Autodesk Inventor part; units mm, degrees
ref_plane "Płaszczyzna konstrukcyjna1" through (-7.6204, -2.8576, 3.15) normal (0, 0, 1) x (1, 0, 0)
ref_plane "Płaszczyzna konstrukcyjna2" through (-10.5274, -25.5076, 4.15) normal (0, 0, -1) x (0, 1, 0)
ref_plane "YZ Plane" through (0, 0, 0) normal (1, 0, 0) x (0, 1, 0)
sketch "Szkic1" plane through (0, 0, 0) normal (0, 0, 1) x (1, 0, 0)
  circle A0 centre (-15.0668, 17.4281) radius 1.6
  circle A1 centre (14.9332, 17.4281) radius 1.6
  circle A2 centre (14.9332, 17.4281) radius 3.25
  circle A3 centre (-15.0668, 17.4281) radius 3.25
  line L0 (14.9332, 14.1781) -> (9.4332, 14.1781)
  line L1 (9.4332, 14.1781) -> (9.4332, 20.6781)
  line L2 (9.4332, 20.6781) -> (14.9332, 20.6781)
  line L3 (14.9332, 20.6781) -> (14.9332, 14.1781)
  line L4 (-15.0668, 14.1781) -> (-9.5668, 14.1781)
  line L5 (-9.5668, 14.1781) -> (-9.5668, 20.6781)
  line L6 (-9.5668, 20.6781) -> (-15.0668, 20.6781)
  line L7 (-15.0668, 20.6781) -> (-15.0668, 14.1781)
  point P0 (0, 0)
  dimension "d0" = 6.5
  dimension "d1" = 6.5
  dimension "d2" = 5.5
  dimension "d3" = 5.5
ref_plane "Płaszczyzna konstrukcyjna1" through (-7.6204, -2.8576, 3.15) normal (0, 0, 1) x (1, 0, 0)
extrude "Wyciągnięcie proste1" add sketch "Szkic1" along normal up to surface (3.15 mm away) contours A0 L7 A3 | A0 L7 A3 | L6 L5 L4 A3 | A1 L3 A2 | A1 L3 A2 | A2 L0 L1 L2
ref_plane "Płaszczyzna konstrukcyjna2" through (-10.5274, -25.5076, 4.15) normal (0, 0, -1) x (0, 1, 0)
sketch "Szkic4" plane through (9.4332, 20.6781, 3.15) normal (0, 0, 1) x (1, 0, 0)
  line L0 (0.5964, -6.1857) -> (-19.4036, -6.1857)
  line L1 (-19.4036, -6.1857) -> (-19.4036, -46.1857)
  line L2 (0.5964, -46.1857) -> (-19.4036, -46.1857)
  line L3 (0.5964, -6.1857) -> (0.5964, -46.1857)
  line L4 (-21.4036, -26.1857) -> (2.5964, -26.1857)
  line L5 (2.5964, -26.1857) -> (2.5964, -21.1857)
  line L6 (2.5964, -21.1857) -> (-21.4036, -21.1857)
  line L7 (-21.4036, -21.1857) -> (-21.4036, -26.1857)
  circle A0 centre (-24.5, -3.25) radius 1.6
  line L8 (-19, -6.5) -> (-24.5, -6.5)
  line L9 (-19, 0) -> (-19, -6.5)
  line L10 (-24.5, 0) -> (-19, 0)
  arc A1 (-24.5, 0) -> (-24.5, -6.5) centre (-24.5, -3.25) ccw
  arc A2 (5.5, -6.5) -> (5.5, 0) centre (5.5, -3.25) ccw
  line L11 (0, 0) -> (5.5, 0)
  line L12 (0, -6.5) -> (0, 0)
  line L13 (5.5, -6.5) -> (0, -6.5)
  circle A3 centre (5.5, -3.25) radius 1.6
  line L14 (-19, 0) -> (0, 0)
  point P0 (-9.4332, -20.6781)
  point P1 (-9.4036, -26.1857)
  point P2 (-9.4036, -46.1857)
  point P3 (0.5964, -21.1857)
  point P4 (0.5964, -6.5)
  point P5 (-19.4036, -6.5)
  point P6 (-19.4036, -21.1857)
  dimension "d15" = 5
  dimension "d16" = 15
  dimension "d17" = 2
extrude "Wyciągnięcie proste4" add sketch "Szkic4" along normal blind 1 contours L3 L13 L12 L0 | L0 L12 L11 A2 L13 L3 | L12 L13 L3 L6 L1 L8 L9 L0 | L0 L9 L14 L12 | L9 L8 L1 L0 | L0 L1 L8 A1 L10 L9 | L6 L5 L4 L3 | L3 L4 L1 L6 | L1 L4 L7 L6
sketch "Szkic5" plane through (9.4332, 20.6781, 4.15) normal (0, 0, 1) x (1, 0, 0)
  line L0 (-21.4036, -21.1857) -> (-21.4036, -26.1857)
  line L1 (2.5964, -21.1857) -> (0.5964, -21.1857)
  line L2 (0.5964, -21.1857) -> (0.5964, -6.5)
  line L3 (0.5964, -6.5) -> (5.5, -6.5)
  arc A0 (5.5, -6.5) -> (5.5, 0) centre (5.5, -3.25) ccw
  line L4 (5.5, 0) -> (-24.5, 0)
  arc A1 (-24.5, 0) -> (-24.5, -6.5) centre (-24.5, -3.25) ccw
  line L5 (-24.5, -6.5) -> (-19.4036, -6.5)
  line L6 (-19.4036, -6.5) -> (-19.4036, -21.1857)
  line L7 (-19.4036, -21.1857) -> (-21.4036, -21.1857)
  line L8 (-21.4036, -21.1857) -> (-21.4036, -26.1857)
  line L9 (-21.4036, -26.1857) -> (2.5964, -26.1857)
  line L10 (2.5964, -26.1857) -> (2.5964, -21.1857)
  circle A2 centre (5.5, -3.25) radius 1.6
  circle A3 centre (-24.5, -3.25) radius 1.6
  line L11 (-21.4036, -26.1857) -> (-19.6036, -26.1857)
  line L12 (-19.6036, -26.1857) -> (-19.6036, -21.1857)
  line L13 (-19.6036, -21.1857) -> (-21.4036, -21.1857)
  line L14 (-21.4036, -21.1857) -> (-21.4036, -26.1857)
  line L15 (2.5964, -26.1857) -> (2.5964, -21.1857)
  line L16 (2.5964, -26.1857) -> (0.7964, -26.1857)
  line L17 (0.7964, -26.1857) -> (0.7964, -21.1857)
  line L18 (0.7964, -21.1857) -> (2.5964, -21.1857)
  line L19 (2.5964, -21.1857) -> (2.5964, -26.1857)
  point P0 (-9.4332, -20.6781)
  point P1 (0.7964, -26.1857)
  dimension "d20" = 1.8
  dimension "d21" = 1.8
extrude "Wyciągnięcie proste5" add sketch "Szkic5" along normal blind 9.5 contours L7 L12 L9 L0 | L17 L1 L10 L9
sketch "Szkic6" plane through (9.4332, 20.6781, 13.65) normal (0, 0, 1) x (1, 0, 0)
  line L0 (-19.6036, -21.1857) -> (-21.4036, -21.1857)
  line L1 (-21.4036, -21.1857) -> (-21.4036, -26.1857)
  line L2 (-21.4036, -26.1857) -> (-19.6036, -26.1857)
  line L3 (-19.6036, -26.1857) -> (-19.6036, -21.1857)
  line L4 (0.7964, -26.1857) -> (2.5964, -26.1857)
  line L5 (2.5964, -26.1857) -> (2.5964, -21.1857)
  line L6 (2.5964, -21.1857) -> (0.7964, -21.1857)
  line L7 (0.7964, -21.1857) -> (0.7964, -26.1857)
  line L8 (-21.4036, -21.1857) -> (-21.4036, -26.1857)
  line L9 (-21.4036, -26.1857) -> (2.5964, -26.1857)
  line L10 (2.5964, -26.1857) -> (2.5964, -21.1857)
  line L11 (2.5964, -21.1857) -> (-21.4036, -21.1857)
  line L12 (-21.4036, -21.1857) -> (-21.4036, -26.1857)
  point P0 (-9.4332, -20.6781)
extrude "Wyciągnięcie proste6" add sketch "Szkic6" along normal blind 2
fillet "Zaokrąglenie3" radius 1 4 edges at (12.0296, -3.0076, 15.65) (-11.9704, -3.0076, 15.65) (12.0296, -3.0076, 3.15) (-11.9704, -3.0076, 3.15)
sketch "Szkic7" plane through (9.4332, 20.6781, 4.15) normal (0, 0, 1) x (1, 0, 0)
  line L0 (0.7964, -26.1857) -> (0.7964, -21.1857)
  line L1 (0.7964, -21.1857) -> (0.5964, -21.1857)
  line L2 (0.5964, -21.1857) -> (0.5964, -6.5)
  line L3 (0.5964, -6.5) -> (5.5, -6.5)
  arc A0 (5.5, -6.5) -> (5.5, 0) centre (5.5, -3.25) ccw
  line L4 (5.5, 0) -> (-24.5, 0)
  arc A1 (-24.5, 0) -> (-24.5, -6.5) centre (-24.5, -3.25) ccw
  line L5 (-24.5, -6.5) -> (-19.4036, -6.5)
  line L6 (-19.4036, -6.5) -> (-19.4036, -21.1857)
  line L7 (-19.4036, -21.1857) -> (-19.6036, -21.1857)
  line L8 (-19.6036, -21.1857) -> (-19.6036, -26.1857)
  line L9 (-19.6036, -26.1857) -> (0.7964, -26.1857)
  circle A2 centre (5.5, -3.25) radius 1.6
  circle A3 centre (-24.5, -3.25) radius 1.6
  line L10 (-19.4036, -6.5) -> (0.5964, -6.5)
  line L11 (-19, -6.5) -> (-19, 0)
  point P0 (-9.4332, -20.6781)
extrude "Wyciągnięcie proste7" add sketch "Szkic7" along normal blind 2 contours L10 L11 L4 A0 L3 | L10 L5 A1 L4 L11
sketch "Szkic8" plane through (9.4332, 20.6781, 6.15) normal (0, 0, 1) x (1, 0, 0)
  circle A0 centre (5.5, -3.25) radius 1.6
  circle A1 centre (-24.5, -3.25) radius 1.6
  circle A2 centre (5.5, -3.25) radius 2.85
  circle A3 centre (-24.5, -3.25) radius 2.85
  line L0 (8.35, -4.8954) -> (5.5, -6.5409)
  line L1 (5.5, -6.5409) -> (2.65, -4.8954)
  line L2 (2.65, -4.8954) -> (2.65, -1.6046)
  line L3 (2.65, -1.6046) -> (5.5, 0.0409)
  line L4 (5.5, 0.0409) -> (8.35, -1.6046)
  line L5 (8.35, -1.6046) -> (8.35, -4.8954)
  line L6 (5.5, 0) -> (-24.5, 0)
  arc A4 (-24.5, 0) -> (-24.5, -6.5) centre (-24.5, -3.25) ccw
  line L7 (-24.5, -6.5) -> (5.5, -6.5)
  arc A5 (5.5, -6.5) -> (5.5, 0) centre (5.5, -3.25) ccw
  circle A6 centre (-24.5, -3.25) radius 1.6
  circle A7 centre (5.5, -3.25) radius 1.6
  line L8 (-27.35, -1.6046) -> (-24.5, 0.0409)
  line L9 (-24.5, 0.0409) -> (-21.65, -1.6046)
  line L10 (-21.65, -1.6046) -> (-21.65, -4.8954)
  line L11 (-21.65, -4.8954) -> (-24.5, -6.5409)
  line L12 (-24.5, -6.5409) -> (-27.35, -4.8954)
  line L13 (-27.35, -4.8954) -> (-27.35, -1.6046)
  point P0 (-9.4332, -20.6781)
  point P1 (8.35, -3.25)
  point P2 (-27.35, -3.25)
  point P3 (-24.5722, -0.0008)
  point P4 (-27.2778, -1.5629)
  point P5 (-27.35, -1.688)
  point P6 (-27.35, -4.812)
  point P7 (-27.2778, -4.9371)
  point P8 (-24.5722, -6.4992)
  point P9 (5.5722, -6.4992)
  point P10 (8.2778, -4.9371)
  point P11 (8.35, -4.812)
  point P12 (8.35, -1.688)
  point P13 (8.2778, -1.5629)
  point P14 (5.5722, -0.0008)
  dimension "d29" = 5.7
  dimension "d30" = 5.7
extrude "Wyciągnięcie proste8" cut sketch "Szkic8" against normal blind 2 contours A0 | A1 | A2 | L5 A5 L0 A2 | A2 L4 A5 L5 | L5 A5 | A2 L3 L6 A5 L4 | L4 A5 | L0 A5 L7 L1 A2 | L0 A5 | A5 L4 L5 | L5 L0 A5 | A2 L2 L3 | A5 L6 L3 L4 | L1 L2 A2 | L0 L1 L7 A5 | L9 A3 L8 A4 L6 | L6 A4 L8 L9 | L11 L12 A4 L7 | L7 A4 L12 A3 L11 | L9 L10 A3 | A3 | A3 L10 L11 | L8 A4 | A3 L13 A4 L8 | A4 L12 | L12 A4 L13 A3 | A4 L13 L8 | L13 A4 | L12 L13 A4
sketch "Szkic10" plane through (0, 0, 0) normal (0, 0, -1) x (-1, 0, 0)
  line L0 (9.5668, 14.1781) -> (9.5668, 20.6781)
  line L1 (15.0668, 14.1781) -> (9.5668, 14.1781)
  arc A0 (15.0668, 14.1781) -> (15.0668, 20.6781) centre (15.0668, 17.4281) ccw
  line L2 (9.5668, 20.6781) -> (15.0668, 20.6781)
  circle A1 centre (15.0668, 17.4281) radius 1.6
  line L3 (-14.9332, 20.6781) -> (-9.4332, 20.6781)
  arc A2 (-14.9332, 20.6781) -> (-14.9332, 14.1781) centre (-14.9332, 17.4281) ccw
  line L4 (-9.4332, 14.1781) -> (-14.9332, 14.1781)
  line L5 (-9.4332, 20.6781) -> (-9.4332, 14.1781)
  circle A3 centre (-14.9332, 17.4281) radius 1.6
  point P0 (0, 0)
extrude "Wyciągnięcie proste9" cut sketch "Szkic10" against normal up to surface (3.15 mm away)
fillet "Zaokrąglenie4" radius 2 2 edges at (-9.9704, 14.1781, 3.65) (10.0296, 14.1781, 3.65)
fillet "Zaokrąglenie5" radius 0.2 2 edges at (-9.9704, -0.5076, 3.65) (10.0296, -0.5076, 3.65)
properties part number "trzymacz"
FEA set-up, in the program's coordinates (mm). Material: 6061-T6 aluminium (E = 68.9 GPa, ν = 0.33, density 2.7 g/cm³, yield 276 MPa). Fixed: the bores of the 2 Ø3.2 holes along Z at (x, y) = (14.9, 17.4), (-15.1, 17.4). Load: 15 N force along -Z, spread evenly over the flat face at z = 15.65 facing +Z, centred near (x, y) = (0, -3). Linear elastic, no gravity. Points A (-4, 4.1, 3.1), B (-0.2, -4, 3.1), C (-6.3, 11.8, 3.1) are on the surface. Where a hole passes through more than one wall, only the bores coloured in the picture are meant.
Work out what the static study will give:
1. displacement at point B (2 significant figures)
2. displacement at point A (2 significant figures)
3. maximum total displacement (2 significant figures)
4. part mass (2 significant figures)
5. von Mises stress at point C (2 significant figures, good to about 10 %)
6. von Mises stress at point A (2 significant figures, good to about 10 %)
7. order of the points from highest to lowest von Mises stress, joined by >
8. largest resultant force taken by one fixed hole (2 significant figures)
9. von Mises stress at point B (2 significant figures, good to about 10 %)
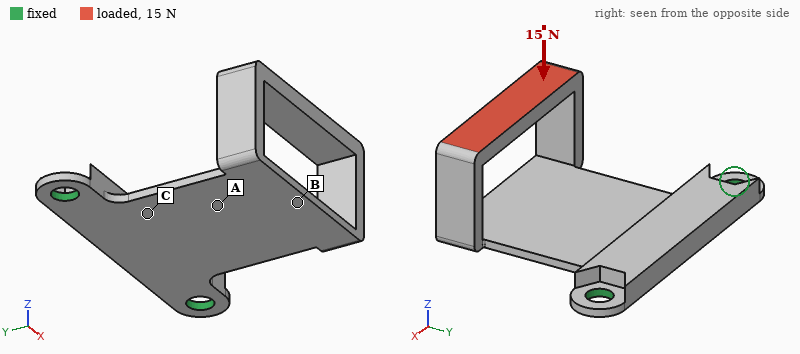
0.29 mm
0.13 mm
0.43 mm
3.7 g
60 MPa
28 MPa
C > A > B
26 N
9.6 MPa
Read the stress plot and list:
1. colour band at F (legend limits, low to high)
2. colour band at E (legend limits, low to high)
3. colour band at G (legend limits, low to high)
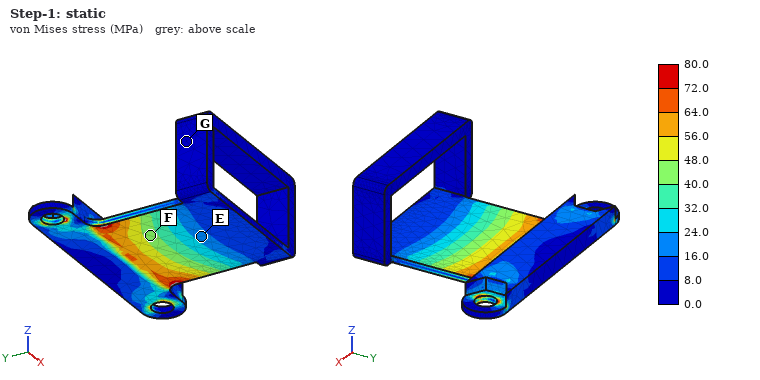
40.0 to 48.0 MPa
16.0 to 24.0 MPa
0.0 to 8.0 MPa
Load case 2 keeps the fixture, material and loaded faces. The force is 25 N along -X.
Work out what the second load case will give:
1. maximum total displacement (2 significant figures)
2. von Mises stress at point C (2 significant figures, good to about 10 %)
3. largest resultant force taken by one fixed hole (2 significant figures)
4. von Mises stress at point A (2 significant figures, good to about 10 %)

0.31 mm
50 MPa
25 N
49 MPa
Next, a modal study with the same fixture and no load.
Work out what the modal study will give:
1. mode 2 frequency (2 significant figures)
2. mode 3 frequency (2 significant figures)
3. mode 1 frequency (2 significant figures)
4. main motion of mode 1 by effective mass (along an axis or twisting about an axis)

1500 Hz
2400 Hz
780 Hz
along Z
